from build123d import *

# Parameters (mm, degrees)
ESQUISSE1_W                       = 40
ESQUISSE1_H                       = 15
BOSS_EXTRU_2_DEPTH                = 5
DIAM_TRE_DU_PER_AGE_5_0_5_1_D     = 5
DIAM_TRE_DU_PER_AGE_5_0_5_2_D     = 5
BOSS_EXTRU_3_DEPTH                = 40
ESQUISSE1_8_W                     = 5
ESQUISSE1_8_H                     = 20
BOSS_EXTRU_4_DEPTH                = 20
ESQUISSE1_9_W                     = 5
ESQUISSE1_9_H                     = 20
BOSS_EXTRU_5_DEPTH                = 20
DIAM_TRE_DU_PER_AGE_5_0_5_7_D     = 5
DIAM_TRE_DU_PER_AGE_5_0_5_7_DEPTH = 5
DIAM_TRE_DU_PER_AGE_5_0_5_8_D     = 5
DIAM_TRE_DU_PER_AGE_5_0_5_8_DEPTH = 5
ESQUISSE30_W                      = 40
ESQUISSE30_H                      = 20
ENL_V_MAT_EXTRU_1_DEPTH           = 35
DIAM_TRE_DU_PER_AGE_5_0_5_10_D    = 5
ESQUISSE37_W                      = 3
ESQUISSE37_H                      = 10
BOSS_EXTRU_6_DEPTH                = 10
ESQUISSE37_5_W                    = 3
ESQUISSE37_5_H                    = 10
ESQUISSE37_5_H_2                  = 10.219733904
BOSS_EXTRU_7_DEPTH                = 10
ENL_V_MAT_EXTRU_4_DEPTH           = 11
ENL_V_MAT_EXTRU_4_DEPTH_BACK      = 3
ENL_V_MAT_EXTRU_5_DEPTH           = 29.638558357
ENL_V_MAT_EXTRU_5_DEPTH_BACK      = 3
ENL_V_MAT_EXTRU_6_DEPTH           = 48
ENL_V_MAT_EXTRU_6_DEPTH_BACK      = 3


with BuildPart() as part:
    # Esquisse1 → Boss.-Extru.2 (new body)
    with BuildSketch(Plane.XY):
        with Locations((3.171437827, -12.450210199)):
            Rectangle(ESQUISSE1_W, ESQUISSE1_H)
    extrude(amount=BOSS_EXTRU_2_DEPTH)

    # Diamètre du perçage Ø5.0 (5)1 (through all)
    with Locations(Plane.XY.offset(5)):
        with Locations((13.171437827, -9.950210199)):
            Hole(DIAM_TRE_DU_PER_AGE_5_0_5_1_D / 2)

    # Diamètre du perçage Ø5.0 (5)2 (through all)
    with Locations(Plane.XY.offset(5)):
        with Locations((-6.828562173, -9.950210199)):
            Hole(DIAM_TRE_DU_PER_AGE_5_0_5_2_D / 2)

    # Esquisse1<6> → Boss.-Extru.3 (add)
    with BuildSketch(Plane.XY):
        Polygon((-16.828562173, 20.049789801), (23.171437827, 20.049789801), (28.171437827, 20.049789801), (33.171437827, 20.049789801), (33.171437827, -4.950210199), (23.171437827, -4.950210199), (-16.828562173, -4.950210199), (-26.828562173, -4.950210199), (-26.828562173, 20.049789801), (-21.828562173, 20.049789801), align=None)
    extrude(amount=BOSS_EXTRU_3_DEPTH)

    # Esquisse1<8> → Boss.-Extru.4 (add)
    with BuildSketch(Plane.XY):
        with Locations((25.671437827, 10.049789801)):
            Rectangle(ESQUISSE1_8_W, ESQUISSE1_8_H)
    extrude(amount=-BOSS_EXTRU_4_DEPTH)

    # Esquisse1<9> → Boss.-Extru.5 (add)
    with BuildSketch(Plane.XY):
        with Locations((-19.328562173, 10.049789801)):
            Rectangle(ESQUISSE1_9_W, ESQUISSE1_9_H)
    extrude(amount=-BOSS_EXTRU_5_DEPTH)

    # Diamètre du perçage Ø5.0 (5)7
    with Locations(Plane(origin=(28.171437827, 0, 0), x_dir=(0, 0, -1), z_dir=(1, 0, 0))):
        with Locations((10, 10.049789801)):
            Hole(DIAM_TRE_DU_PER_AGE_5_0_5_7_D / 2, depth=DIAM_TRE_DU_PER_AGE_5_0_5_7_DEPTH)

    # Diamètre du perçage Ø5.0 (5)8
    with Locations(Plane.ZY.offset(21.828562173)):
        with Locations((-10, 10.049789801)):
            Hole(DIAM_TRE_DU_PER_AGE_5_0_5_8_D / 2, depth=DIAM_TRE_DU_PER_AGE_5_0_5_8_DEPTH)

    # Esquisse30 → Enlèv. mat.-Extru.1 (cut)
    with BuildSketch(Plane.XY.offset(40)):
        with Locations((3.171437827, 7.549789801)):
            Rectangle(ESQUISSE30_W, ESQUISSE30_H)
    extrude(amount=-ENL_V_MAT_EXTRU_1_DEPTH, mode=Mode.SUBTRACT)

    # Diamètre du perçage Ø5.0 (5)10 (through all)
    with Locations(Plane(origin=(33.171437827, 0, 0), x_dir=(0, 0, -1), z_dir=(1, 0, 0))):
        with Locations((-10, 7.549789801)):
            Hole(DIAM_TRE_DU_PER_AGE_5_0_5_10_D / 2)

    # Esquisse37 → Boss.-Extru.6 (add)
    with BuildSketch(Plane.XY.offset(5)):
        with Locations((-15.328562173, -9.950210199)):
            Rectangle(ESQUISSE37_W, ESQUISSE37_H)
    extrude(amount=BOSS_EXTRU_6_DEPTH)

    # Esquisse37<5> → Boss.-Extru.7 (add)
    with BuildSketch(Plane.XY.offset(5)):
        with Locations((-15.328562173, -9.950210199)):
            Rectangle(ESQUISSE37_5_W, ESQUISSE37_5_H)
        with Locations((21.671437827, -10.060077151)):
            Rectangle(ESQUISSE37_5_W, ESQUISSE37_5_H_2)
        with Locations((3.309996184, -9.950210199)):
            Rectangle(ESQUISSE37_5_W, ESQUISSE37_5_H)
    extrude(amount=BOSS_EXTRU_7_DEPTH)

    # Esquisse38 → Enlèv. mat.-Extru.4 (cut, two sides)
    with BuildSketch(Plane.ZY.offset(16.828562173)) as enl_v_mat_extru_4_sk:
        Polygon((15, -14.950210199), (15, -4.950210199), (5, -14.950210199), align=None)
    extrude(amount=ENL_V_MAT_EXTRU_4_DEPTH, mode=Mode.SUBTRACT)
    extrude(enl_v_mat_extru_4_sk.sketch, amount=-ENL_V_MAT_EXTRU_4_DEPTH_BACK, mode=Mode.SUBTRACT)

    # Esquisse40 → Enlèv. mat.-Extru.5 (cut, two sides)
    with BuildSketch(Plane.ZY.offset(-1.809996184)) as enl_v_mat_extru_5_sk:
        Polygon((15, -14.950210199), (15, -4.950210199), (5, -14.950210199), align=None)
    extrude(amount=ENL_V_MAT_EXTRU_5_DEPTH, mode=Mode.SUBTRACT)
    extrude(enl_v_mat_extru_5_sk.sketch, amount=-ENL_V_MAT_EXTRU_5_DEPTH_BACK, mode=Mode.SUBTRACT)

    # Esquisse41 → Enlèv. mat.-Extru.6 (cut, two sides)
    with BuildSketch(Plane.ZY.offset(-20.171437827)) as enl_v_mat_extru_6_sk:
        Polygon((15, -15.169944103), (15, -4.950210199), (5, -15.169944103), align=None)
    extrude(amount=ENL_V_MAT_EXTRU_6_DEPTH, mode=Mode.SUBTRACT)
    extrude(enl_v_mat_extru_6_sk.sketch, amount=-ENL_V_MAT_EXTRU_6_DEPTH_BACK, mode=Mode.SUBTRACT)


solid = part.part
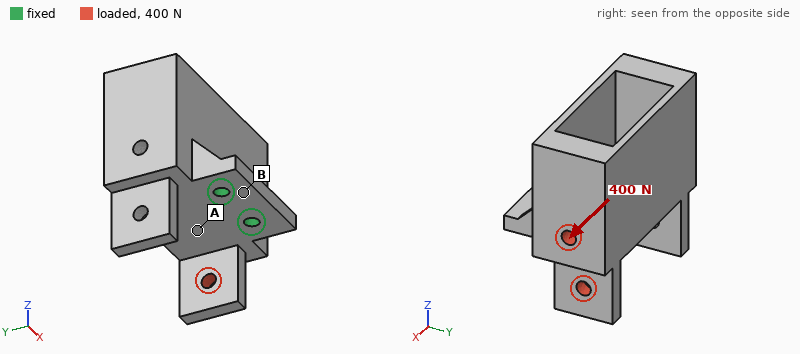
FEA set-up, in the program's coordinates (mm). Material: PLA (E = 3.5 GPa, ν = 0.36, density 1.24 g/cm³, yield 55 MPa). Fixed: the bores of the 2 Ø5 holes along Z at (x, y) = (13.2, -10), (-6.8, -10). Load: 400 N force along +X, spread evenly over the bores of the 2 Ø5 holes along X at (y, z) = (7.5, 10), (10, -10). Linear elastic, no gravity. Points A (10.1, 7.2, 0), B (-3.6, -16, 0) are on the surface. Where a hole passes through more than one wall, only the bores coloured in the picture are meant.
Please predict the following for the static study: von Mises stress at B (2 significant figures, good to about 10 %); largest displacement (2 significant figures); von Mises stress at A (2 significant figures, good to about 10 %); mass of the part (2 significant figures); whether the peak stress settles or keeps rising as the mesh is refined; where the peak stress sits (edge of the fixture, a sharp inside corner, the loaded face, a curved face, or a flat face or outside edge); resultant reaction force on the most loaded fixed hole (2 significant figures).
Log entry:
1.8 MPa
0.32 mm
3.6 MPa
48 g
keeps rising
edge of the fixture
370 N
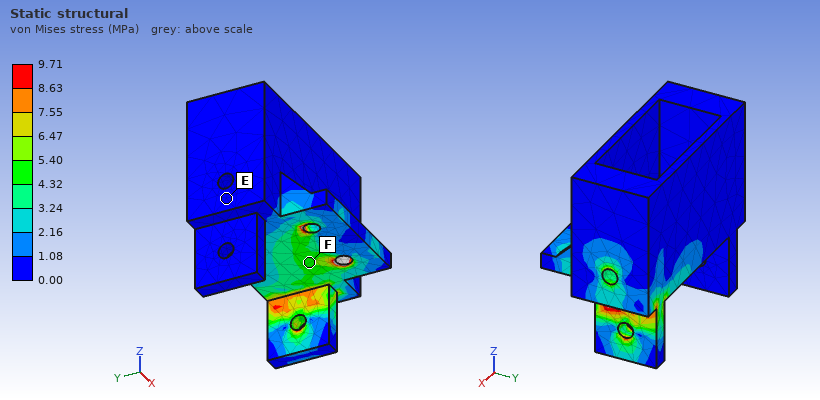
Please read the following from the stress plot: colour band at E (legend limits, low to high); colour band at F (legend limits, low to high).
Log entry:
0.00 to 1.08 MPa
4.32 to 5.40 MPa
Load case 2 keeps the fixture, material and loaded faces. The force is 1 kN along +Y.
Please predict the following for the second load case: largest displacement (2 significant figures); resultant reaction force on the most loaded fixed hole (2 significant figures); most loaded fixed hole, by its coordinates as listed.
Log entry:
0.34 mm
1.5 kN
(13.2, -10)
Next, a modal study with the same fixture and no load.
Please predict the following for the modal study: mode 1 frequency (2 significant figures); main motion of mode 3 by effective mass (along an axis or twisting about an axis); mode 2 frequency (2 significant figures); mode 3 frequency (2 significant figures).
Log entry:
500 Hz
along X
820 Hz
1600 Hz
